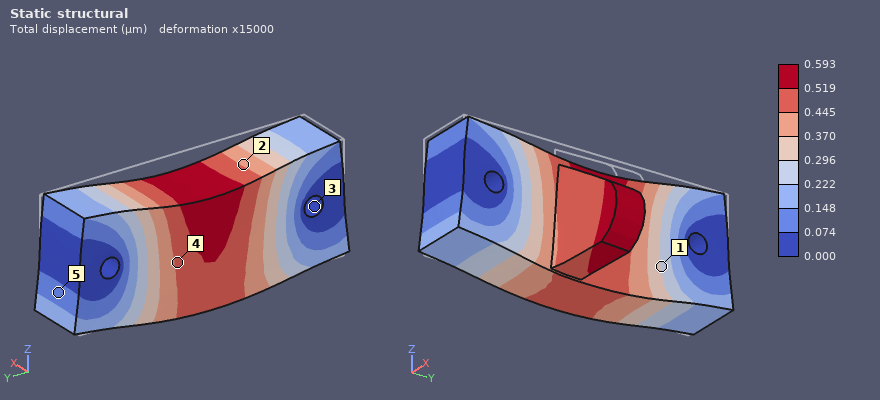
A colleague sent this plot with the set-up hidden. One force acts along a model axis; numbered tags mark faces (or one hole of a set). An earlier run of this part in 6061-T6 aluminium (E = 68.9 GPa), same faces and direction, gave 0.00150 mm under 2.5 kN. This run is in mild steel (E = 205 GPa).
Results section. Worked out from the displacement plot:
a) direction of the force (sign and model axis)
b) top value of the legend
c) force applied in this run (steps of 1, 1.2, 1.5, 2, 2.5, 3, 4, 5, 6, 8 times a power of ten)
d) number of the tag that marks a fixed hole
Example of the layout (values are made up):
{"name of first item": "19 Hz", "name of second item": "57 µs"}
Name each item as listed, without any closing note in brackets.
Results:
{"direction of the force": "-Z", "top value of the legend": "0.593 µm", "force applied in this run": "3 kN", "number of the tag that marks a fixed hole": "3"}
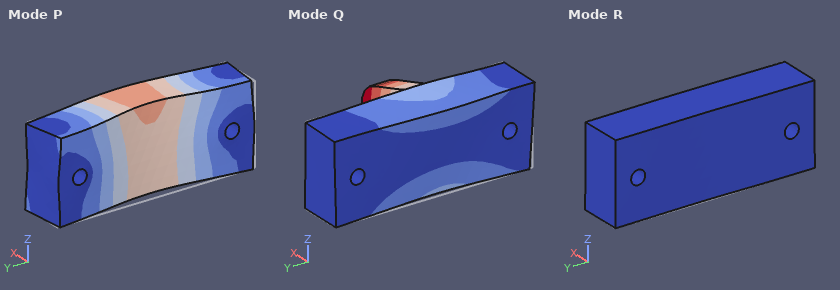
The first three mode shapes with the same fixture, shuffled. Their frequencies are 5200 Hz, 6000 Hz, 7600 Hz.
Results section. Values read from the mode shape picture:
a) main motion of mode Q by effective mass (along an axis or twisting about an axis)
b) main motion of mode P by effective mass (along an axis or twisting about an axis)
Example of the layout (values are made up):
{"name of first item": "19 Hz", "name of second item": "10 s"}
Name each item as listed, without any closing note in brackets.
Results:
{"main motion of mode Q by effective mass": "along Z", "main motion of mode P by effective mass": "along X"}
